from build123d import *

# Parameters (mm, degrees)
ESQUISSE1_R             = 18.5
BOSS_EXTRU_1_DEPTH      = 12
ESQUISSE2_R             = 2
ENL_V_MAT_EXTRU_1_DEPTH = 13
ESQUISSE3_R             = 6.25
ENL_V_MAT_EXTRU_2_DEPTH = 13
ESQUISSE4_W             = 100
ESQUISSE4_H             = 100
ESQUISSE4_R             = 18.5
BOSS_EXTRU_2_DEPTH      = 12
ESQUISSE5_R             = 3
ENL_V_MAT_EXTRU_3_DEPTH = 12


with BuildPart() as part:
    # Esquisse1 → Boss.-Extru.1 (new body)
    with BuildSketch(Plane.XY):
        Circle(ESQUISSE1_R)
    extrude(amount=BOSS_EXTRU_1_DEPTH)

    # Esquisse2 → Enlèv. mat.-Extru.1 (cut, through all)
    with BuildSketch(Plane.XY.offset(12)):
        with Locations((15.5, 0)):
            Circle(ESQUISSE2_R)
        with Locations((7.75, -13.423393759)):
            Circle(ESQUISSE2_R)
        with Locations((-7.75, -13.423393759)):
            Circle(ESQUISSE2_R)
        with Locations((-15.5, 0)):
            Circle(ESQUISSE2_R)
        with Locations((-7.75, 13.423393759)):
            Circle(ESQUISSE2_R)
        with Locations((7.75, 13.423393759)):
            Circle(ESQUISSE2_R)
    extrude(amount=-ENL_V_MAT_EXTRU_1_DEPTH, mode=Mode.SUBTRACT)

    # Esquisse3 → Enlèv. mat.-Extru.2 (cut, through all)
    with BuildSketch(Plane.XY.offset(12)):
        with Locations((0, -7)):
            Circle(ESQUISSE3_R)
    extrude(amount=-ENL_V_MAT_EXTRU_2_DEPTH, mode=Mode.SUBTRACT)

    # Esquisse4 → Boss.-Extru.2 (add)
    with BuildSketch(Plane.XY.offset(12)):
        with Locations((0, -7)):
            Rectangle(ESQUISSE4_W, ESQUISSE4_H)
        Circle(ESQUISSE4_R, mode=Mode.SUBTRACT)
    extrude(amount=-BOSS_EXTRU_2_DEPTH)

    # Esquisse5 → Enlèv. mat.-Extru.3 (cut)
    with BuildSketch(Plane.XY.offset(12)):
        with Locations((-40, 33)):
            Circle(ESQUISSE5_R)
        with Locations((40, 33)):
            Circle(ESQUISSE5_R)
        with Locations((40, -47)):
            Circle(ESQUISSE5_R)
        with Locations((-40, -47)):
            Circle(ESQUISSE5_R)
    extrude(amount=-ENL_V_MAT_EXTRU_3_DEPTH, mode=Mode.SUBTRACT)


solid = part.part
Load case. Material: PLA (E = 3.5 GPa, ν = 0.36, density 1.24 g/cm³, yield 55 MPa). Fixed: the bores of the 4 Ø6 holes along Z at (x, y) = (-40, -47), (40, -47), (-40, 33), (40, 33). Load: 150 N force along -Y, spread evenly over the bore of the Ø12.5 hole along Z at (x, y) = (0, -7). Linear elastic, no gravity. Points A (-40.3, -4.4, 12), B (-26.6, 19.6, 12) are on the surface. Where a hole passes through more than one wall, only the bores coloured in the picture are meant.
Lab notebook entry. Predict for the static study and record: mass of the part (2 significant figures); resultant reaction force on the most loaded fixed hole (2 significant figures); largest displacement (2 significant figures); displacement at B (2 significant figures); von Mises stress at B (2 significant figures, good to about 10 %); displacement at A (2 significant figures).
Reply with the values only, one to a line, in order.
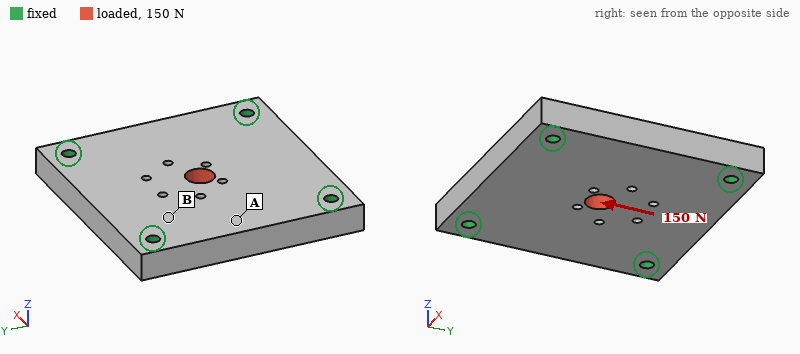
140 g
42 N
3.6 µm
1.1 µm
0.16 MPa
0.73 µm
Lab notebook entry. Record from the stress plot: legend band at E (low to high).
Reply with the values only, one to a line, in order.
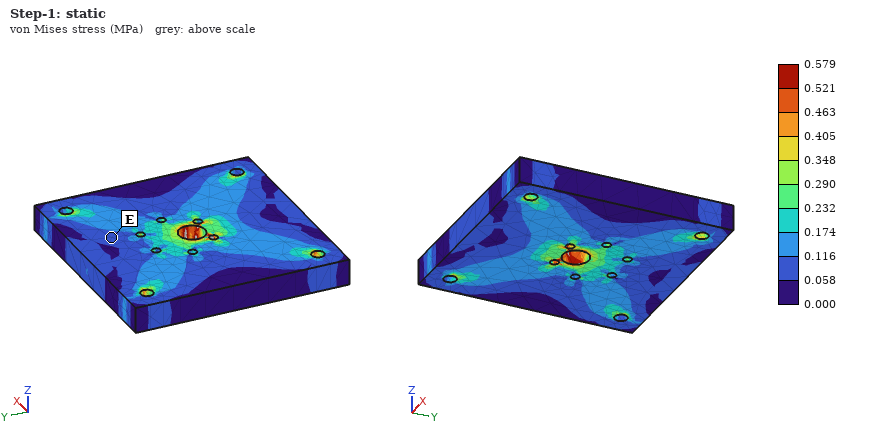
0.058 to 0.116 MPa
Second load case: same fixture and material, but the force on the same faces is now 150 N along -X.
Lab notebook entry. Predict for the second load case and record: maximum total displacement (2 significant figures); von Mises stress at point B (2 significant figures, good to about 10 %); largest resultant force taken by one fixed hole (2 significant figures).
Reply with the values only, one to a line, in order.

3.7 µm
0.16 MPa
43 N
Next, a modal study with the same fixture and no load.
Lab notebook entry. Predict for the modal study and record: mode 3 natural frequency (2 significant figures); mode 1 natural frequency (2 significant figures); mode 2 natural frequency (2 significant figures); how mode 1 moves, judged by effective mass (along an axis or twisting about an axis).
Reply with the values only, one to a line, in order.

3000 Hz
1900 Hz
3000 Hz
along Z
